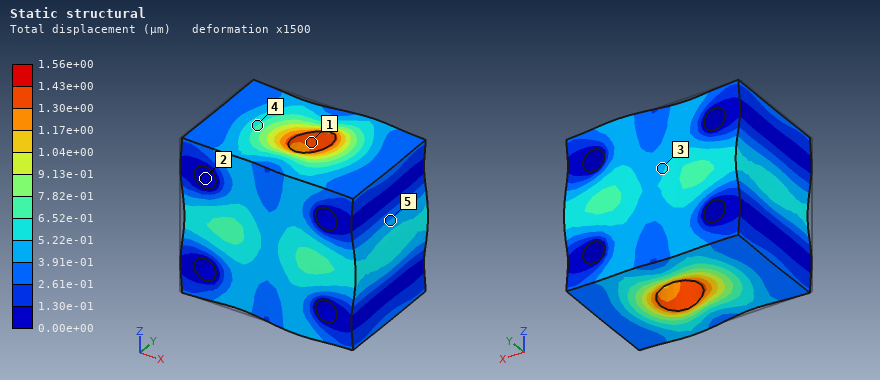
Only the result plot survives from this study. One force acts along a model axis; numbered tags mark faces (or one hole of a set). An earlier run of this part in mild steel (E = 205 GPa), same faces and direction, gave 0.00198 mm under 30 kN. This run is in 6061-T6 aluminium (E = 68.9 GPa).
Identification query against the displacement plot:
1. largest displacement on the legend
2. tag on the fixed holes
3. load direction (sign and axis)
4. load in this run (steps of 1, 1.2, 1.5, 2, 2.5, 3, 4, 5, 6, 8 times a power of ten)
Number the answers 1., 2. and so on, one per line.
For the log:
1. 1.56e+00 µm
2. 2
3. +X
4. 8 kN
